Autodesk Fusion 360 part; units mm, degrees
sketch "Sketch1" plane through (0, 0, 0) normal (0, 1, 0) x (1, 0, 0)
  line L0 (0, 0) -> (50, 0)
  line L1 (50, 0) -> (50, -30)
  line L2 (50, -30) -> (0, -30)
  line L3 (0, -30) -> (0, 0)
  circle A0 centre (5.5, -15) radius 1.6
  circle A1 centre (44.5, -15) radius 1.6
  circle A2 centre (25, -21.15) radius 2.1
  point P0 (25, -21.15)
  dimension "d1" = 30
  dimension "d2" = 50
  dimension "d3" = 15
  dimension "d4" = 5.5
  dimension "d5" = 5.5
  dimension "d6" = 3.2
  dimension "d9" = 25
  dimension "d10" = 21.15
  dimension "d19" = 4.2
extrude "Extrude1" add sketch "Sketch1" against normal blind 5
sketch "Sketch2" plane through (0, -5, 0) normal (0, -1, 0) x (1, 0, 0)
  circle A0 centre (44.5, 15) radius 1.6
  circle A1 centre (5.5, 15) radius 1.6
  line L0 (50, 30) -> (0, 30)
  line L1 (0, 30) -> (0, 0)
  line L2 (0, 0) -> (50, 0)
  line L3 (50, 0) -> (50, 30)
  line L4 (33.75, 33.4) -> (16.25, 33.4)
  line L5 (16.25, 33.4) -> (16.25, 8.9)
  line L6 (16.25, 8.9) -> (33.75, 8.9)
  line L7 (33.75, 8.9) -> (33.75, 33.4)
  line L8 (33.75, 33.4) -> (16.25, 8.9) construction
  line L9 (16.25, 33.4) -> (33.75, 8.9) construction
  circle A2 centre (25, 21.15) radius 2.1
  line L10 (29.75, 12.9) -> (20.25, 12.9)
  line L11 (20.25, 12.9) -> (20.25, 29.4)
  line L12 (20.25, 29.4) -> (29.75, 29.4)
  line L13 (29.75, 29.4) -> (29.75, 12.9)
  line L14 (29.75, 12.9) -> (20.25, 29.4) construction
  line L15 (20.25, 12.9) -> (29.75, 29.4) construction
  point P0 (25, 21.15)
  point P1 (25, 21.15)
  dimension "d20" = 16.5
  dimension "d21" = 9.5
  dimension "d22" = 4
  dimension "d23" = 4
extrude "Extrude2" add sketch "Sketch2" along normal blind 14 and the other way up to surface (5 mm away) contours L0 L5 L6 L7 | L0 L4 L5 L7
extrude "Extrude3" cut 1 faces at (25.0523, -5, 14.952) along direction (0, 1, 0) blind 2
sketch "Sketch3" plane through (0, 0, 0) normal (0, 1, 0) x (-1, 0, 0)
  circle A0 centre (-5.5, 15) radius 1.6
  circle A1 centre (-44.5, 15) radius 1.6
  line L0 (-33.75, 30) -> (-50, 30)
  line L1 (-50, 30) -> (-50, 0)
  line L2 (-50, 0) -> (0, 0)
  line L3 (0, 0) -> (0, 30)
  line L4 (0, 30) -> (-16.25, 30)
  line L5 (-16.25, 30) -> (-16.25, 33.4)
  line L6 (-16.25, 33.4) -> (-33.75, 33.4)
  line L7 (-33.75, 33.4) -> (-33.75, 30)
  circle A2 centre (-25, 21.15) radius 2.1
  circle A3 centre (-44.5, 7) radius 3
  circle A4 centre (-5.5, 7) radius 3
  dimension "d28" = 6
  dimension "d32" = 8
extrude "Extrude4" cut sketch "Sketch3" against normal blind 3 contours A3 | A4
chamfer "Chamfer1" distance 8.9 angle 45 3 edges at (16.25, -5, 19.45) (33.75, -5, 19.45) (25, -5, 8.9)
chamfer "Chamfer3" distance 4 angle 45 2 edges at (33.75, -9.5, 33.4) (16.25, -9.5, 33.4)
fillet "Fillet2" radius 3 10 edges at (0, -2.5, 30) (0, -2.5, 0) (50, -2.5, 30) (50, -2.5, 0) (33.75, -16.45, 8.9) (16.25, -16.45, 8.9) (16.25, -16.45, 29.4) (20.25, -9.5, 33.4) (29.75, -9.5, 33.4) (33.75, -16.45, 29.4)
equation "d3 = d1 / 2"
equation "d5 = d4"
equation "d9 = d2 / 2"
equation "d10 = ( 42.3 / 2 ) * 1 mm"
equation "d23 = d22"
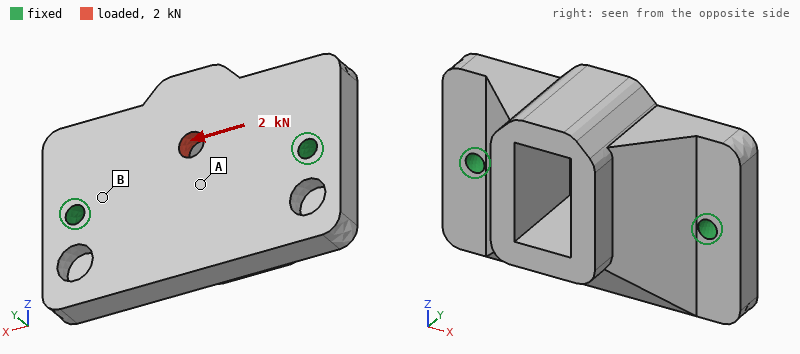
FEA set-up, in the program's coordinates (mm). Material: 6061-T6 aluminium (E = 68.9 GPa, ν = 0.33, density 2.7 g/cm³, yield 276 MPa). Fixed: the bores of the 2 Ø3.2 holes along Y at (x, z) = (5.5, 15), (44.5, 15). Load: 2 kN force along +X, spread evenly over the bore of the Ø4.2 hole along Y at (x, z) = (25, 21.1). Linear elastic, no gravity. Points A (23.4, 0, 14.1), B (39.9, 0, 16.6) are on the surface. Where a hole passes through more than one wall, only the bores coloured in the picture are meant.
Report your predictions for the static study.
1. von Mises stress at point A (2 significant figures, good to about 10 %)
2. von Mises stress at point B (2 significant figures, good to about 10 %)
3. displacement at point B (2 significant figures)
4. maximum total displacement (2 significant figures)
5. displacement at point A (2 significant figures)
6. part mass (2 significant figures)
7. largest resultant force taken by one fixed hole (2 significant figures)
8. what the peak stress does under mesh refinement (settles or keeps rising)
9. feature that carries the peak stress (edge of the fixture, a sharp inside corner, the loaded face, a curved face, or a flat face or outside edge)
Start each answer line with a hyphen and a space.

- 9.1 MPa
- 24 MPa
- 1.2 µm
- 7.7 µm
- 2.7 µm
- 36 g
- 1.0 kN
- keeps rising
- edge of the fixture
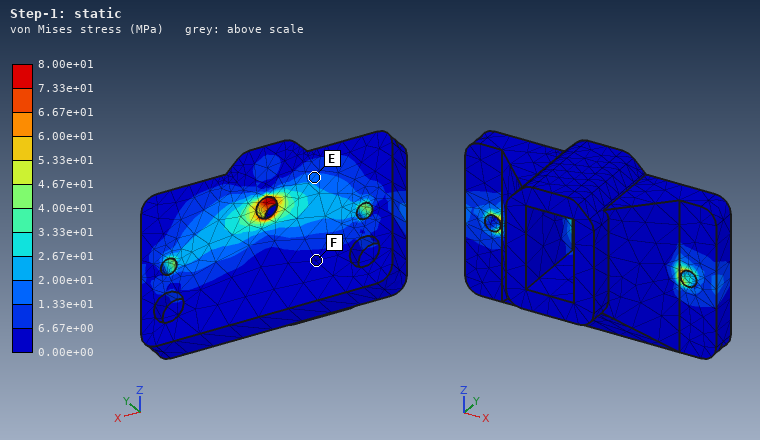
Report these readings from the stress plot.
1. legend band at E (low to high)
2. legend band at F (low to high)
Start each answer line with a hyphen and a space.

- 1.33e+01 to 2.00e+01 MPa
- 0.00e+00 to 6.67e+00 MPa
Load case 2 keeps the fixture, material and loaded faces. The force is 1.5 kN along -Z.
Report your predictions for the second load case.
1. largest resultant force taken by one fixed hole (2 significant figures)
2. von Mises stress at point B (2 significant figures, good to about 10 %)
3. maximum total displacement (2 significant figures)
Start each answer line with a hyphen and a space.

- 750 N
- 14 MPa
- 8.5 µm
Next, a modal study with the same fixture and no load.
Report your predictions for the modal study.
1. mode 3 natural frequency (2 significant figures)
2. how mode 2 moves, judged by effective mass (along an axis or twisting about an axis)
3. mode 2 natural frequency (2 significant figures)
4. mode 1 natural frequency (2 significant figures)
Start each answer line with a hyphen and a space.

- 22 kHz
- along Y
- 14 kHz
- 6300 Hz
